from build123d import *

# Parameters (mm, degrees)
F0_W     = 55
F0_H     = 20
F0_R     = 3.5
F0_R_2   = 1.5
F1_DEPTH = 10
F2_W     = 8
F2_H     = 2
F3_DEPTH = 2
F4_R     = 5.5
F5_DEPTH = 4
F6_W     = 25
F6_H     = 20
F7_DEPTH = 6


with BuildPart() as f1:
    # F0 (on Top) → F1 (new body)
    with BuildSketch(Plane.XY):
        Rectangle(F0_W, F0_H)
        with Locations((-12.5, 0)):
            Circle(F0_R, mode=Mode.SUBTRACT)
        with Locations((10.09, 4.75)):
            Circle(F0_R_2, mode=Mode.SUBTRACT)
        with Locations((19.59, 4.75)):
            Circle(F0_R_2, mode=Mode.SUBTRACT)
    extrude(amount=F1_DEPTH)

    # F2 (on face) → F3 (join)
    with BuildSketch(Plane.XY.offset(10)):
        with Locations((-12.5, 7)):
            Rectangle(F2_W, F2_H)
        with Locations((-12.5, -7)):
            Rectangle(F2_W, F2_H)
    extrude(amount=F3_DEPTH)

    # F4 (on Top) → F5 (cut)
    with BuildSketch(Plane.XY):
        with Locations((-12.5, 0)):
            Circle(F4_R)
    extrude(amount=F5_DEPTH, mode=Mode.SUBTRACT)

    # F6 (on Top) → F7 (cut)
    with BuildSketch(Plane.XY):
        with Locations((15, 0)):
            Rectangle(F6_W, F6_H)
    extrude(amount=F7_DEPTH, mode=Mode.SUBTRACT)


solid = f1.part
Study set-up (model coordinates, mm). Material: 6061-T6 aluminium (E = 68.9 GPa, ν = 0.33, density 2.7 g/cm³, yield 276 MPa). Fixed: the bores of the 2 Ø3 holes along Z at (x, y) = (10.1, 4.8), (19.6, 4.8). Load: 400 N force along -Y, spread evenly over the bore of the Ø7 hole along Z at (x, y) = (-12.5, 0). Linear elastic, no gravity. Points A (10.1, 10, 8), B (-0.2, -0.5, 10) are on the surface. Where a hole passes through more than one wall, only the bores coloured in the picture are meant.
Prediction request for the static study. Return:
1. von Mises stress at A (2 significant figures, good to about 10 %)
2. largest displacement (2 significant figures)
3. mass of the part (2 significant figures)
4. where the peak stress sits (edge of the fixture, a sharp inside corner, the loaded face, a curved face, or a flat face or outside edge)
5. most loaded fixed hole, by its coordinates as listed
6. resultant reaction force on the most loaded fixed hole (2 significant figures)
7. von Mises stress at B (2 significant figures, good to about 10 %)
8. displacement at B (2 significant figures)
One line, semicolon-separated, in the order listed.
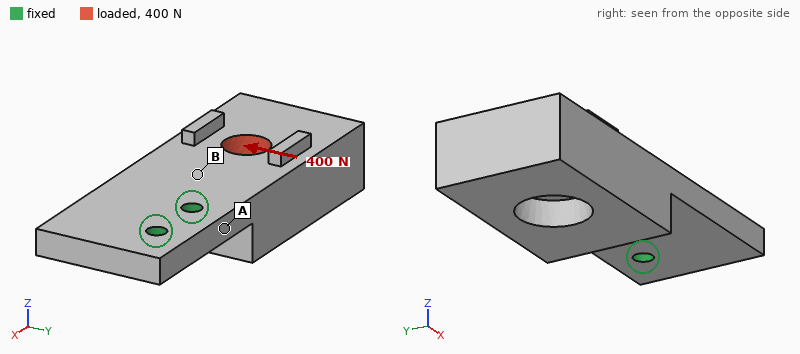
43 MPa; 48 µm; 20 g; edge of the fixture; (10.1, 4.8); 1.1 kN; 14 MPa; 12 µm
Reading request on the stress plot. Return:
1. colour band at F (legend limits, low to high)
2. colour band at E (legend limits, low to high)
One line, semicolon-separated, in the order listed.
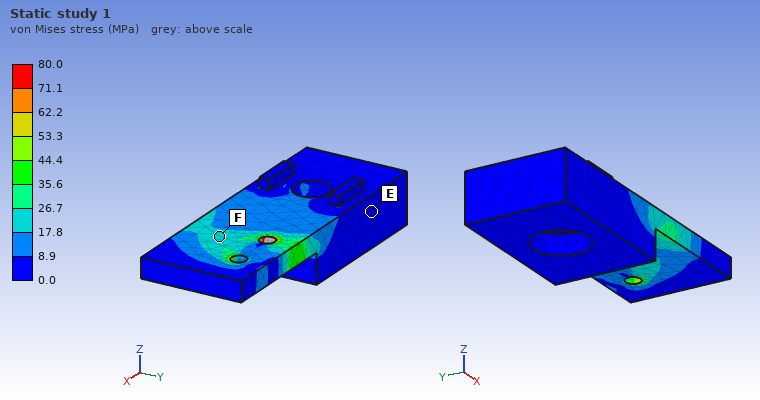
17.8 to 26.7 MPa; 0.0 to 8.9 MPa
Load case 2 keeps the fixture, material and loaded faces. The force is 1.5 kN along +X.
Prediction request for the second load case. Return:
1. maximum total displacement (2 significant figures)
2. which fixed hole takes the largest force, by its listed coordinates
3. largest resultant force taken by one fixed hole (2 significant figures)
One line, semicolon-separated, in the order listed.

71 µm; (10.1, 4.8); 1.2 kN
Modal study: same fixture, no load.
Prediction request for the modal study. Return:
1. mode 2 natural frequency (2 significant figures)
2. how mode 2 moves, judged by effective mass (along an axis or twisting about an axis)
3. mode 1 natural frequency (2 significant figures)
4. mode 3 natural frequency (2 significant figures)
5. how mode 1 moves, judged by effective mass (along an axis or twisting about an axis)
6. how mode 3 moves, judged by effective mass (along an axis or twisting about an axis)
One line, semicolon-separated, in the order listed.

4300 Hz; along Y; 1600 Hz; 6100 Hz; along Z; twisting about X
